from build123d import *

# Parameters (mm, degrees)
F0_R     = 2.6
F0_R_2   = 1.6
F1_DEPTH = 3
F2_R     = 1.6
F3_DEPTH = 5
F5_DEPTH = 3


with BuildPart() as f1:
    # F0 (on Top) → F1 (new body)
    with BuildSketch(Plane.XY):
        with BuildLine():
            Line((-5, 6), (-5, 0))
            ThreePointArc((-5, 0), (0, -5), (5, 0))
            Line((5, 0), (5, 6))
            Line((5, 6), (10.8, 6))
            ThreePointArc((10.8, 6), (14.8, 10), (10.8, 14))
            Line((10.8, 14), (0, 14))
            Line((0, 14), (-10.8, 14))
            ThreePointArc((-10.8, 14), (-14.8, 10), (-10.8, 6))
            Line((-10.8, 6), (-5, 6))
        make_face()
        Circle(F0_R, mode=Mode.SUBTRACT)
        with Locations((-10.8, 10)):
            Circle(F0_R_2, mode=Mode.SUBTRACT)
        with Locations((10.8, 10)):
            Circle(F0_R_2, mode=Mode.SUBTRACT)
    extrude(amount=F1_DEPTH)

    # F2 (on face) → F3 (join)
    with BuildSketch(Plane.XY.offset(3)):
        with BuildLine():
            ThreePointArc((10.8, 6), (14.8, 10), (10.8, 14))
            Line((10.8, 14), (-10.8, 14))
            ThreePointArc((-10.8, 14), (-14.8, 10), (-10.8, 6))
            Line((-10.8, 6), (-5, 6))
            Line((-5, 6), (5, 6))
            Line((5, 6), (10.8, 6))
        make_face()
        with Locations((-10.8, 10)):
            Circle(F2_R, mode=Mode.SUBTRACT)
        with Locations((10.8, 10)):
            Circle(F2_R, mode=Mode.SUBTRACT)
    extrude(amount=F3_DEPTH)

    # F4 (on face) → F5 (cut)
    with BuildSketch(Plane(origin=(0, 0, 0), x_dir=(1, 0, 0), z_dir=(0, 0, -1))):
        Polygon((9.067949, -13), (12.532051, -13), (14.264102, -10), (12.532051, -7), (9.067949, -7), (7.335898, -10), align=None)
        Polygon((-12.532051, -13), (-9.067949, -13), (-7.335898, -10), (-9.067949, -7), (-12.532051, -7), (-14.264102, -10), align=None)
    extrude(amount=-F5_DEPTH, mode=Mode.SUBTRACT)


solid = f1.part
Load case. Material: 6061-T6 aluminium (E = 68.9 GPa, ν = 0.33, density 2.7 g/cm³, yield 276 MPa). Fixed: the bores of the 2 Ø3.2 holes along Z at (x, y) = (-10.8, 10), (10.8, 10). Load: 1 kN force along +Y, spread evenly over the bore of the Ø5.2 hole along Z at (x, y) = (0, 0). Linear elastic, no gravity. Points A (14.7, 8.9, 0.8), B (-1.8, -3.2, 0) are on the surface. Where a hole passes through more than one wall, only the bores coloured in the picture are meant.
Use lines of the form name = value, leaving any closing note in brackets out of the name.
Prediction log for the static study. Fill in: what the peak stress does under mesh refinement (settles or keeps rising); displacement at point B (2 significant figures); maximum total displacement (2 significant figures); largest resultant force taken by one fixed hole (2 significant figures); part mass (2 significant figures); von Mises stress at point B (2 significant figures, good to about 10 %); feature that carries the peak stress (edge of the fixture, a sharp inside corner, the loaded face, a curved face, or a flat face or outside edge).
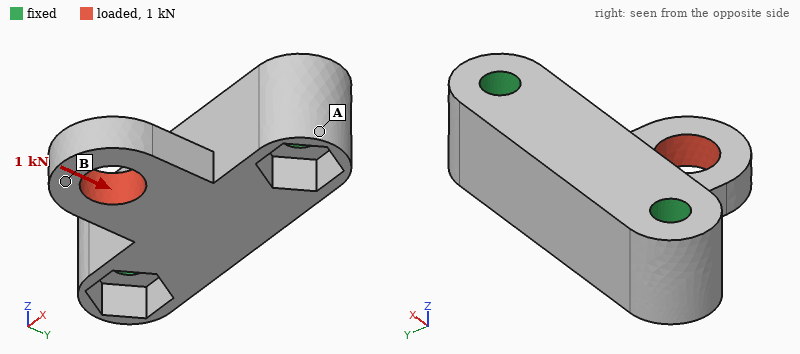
what the peak stress does under mesh refinement = keeps rising
displacement at point B = 29 µm
maximum total displacement = 32 µm
largest resultant force taken by one fixed hole = 500 N
part mass = 4.7 g
von Mises stress at point B = 32 MPa
feature that carries the peak stress = edge of the fixture
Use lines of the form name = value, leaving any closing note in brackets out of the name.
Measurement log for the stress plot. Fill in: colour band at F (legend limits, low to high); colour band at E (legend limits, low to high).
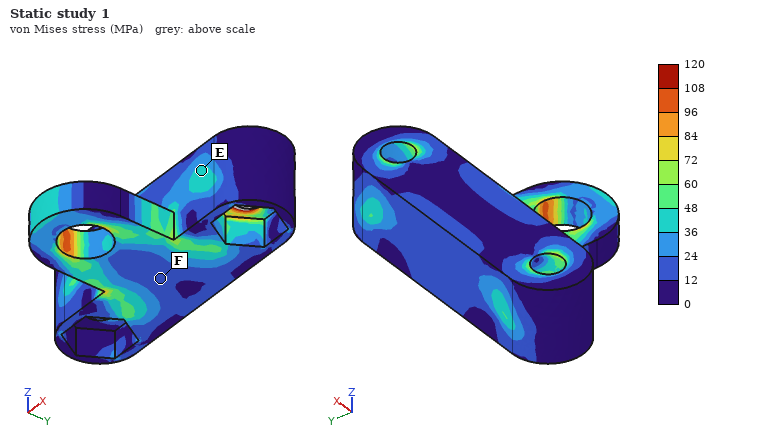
colour band at F = 12 to 24 MPa
colour band at E = 36 to 48 MPa
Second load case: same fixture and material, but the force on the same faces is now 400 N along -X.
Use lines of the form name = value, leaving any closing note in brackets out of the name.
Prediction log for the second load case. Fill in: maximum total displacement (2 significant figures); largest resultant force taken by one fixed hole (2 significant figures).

maximum total displacement = 24 µm
largest resultant force taken by one fixed hole = 300 N
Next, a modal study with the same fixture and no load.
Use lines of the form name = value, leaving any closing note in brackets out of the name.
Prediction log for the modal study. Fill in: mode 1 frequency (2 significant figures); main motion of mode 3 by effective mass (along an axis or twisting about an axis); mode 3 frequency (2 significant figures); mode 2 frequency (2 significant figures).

mode 1 frequency = 16 kHz
main motion of mode 3 by effective mass = along Y
mode 3 frequency = 36 kHz
mode 2 frequency = 33 kHz
